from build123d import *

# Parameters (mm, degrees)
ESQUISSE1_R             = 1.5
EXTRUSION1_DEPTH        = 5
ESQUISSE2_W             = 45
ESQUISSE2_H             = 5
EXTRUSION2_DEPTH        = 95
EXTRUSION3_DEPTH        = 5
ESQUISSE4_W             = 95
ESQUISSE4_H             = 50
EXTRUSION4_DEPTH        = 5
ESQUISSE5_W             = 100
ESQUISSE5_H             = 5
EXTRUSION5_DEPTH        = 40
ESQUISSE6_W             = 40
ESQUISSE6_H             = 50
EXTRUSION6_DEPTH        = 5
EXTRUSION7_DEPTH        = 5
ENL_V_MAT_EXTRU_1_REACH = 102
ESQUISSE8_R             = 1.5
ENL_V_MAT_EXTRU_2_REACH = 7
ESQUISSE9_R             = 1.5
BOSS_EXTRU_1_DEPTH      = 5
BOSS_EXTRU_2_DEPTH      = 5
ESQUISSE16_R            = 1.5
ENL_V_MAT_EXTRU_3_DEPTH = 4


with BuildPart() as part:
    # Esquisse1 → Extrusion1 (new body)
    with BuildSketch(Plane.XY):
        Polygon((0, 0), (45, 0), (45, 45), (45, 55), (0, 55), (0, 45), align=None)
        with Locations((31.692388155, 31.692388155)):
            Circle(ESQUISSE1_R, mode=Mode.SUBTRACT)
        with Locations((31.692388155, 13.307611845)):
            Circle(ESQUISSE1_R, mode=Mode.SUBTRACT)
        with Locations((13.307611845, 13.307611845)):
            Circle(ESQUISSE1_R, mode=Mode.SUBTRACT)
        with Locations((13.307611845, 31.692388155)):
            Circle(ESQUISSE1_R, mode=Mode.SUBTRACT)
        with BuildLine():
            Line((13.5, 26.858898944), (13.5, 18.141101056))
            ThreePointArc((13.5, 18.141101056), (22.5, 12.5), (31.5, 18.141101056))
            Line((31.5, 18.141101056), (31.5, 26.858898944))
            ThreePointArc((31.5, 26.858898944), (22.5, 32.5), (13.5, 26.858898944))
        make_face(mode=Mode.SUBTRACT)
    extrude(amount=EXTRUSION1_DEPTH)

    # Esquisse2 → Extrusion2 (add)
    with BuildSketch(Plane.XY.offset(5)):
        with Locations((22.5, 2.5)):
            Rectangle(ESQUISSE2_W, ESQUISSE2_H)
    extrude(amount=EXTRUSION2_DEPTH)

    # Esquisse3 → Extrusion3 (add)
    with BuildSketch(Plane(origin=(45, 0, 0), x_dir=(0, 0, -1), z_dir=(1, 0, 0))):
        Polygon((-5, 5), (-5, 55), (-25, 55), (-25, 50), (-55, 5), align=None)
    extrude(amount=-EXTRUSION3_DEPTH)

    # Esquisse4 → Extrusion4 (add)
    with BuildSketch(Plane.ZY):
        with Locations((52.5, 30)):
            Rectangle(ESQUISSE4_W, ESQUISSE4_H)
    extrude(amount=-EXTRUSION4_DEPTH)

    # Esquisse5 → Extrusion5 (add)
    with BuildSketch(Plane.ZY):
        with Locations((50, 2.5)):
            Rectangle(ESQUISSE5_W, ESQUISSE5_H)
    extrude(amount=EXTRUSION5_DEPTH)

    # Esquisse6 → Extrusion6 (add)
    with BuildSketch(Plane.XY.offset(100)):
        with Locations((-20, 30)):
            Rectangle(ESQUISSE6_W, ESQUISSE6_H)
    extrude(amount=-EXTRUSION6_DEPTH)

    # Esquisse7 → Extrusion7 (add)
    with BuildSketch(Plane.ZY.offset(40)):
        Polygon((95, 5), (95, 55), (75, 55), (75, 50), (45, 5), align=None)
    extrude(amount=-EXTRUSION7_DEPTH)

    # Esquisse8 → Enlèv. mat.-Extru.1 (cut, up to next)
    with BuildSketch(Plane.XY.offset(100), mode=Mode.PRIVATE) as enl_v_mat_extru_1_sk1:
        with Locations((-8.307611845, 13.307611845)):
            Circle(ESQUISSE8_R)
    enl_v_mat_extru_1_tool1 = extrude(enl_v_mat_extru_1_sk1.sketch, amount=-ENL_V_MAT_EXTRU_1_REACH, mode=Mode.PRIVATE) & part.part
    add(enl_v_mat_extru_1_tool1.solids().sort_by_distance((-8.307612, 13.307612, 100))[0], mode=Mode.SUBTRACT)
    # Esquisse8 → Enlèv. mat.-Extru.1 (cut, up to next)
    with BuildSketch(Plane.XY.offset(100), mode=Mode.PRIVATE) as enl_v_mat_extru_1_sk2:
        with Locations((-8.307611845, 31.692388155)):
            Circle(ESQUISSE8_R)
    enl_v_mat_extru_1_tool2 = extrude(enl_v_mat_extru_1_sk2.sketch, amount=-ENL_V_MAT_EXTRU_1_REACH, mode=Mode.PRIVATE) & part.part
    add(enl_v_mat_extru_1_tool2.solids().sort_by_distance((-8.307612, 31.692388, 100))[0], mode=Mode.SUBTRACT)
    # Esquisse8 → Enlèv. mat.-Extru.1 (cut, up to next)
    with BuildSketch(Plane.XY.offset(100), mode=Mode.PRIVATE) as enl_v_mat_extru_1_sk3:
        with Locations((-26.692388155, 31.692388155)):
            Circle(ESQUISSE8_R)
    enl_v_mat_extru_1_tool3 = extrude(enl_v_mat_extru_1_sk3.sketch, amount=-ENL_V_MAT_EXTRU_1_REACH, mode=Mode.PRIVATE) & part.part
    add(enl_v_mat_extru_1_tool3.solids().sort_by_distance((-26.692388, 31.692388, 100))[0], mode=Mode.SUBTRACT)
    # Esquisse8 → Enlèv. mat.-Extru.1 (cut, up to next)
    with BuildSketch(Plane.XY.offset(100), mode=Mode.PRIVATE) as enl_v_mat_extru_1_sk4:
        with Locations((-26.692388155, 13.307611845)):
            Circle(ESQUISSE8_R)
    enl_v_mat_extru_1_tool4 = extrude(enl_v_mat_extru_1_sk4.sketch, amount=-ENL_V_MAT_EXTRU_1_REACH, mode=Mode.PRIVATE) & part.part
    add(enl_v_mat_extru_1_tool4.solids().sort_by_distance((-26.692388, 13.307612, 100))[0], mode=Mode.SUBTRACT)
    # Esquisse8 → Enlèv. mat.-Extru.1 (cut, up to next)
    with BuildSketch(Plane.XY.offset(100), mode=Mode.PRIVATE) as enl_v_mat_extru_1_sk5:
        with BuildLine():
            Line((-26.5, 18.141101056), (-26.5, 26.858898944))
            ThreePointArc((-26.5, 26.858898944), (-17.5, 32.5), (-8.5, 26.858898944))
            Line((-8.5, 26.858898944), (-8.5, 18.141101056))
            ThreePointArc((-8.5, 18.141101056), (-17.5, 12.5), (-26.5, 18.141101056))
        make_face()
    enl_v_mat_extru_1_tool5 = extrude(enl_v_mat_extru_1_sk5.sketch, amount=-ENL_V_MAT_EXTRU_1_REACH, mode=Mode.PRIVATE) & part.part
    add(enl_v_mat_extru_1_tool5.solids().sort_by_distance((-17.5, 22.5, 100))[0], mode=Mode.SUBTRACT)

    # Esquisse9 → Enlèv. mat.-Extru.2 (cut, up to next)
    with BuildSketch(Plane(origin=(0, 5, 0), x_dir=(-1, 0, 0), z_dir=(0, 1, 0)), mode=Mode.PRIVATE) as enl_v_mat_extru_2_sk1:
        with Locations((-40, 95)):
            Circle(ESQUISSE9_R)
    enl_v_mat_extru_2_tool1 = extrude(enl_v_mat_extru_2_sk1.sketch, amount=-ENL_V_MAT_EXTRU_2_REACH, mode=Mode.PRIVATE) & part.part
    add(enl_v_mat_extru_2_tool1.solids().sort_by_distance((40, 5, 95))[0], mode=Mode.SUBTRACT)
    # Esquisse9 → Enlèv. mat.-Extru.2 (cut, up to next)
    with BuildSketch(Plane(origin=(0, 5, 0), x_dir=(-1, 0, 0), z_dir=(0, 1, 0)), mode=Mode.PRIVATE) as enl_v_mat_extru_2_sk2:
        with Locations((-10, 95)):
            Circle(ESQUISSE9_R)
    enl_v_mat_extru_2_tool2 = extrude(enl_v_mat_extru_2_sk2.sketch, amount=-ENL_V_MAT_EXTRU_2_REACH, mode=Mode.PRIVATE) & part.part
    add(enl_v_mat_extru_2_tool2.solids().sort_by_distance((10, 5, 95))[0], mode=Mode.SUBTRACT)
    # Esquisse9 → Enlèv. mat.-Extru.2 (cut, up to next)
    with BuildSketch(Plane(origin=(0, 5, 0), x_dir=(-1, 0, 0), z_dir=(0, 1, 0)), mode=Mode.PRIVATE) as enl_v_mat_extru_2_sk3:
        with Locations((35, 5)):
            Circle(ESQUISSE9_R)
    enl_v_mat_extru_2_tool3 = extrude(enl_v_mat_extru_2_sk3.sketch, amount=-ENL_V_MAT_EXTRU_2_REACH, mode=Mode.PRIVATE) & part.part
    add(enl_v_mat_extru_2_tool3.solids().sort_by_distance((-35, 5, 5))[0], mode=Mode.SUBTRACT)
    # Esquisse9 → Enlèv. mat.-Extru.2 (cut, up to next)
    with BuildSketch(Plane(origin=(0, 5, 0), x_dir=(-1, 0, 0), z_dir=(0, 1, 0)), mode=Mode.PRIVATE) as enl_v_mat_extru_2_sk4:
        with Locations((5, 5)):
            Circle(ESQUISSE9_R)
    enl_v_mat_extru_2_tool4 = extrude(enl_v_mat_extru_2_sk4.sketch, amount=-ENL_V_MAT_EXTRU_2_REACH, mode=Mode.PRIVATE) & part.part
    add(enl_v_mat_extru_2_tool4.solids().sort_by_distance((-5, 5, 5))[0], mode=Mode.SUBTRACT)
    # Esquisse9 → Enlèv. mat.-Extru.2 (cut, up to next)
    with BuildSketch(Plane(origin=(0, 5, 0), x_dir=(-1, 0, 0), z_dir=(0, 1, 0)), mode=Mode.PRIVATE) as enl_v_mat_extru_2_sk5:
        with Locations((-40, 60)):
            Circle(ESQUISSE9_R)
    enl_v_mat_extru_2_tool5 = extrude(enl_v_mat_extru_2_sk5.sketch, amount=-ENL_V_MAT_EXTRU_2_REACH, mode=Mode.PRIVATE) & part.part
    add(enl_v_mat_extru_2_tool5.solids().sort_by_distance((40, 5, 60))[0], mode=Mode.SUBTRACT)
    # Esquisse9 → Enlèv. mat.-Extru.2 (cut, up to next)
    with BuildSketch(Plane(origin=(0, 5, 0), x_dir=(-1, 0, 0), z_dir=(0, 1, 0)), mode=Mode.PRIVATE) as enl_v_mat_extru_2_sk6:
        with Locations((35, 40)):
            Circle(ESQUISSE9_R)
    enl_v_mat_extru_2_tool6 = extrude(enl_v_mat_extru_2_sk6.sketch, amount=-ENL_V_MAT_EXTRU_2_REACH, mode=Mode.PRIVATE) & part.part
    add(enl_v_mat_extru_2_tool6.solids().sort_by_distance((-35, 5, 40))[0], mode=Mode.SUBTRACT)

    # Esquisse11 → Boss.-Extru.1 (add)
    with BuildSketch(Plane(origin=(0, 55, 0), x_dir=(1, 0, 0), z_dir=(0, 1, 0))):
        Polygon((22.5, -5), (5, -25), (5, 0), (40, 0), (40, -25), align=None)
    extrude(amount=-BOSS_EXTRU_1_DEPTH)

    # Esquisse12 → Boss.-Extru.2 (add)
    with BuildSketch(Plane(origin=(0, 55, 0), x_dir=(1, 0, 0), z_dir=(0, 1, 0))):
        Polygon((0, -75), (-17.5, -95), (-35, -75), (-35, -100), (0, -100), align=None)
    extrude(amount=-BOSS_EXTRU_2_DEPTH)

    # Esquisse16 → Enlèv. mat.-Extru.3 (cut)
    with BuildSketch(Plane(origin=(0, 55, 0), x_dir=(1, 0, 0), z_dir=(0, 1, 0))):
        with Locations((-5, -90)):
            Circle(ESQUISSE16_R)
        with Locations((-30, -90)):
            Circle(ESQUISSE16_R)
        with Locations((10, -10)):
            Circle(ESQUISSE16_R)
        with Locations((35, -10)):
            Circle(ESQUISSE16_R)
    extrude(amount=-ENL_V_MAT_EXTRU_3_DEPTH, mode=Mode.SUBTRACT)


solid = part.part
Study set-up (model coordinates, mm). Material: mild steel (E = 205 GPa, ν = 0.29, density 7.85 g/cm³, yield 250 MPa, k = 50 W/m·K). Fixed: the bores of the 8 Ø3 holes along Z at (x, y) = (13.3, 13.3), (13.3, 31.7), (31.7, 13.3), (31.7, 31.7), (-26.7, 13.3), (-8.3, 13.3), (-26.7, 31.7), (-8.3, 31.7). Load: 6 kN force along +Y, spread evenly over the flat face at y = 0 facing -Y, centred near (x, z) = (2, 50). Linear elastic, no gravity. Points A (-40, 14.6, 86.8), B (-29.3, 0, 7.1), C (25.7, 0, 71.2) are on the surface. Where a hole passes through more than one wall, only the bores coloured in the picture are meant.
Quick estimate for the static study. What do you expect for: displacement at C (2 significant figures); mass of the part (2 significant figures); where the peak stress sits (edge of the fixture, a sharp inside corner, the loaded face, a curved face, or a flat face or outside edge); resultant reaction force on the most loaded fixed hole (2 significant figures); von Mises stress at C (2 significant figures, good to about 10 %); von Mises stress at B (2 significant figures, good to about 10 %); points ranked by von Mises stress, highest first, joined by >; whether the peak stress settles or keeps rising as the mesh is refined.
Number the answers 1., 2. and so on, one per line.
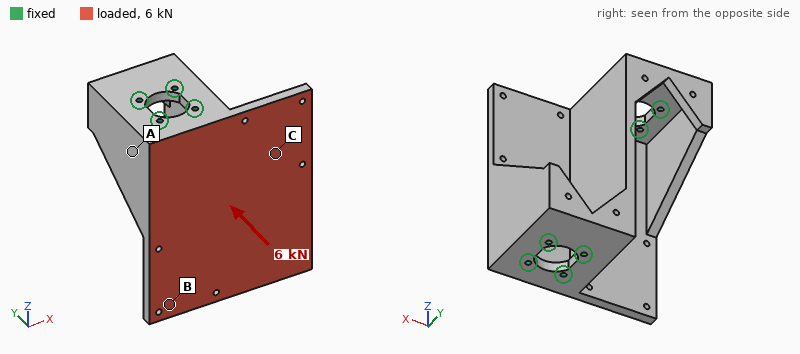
1. 26 µm
2. 820 g
3. edge of the fixture
4. 1.2 kN
5. 34 MPa
6. 22 MPa
7. C > B > A
8. keeps rising
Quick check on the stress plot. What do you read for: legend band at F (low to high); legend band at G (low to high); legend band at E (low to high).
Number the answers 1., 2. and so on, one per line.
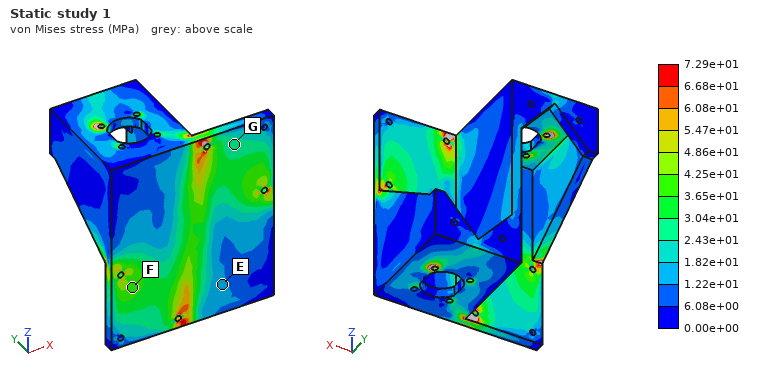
1. 3.65e+01 to 4.25e+01 MPa
2. 2.43e+01 to 3.04e+01 MPa
3. 1.22e+01 to 1.82e+01 MPa
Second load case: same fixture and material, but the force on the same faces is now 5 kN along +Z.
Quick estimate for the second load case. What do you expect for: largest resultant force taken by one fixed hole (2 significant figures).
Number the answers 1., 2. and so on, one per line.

1. 1.3 kN
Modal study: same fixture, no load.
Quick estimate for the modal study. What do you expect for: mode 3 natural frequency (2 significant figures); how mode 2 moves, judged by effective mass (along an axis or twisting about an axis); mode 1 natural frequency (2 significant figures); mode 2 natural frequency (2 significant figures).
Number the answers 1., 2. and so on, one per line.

1. 4100 Hz
2. along Y
3. 3000 Hz
4. 3300 Hz
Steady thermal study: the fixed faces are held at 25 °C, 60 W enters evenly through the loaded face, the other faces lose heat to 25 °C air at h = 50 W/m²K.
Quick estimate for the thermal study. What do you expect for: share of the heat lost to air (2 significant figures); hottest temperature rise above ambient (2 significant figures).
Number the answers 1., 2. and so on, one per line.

1. 43 %
2. 36 K
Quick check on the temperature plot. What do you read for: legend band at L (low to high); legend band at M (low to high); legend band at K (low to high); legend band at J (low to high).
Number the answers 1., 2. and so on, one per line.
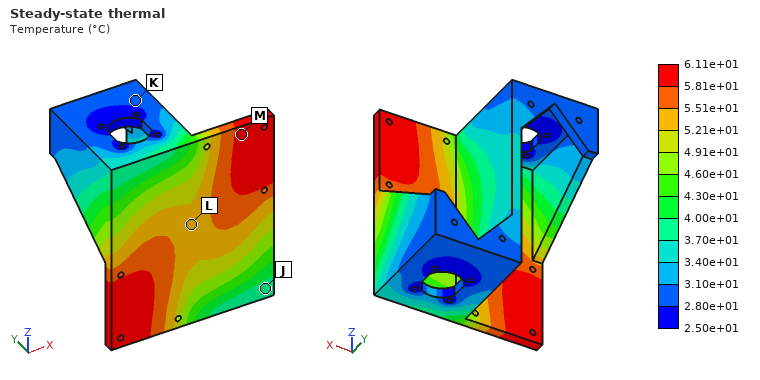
1. 5.21e+01 to 5.51e+01 °C
2. 5.81e+01 to 6.11e+01 °C
3. 2.80e+01 to 3.10e+01 °C
4. 3.70e+01 to 4.00e+01 °C
